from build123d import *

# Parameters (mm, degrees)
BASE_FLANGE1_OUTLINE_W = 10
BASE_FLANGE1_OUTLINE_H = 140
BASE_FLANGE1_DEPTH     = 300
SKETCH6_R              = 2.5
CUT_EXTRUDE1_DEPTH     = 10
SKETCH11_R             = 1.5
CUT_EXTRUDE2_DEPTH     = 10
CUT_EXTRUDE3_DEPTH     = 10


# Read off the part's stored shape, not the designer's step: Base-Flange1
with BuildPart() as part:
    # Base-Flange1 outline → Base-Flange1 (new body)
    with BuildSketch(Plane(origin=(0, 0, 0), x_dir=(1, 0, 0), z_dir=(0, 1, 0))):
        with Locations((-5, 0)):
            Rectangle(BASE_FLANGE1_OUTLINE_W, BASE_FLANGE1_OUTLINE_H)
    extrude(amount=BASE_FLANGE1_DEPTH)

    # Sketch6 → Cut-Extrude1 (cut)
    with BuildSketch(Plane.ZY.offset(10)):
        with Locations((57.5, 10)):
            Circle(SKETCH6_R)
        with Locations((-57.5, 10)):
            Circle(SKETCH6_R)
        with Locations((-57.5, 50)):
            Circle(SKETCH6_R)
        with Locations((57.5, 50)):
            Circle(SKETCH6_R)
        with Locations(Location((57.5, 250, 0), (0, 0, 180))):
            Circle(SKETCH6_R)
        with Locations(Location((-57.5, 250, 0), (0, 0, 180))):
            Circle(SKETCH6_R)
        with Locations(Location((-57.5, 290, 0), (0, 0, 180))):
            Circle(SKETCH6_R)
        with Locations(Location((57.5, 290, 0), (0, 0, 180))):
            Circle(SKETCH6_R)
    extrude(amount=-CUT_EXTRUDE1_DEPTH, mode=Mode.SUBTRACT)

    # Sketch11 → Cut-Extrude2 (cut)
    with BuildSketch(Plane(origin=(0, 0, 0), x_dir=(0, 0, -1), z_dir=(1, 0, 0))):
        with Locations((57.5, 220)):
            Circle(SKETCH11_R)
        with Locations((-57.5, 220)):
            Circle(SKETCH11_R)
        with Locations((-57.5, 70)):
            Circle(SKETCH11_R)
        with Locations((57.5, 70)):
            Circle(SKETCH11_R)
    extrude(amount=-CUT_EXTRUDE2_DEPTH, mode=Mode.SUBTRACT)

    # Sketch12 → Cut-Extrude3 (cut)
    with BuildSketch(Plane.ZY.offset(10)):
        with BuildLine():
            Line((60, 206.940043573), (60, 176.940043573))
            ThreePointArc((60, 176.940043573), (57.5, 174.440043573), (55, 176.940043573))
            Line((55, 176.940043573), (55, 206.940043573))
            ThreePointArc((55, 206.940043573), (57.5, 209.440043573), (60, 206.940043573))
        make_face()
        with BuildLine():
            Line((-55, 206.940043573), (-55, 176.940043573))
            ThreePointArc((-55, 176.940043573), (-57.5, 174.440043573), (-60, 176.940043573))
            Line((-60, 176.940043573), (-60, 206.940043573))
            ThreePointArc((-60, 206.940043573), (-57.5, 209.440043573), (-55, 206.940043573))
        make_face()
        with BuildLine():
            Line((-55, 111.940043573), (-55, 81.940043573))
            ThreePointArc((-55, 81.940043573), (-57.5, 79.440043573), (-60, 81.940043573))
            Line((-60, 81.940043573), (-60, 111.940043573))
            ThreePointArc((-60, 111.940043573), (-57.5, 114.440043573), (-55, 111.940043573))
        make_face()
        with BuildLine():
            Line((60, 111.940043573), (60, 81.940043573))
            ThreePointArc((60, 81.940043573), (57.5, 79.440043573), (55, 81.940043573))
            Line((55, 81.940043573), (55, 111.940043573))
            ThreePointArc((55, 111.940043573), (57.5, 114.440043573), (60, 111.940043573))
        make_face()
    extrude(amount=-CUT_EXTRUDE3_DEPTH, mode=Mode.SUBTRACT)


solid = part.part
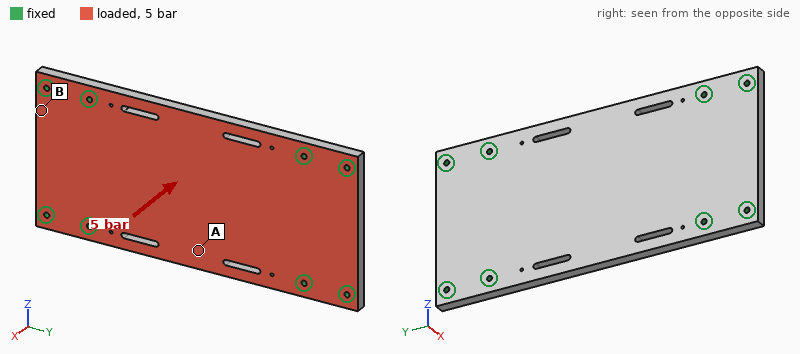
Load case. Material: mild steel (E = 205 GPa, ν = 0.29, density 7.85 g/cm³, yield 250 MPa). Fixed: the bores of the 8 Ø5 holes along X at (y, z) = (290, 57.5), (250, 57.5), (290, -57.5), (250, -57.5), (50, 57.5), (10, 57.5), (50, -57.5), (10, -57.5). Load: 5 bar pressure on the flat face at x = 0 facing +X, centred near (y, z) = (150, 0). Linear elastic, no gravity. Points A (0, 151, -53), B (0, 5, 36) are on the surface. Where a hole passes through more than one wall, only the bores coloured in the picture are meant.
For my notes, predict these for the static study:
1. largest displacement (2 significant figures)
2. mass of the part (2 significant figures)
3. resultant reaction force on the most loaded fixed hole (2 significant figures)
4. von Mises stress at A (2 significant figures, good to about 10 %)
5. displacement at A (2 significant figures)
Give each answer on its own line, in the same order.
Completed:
0.18 mm
3.2 kg
5.3 kN
56 MPa
0.17 mm
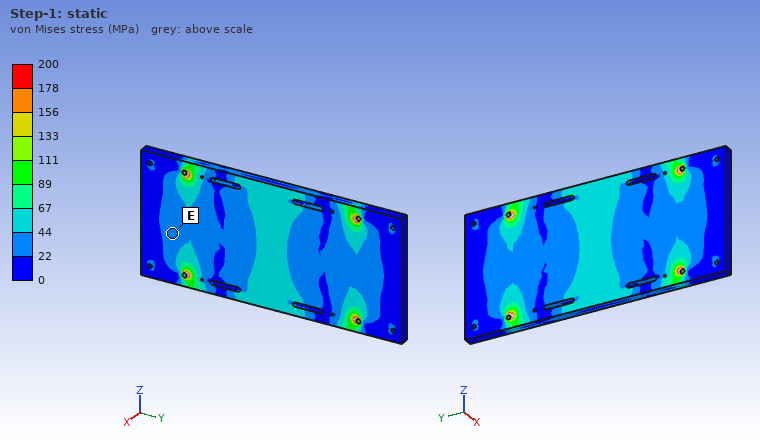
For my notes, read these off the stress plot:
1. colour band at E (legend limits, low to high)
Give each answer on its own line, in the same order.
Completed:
22 to 44 MPa
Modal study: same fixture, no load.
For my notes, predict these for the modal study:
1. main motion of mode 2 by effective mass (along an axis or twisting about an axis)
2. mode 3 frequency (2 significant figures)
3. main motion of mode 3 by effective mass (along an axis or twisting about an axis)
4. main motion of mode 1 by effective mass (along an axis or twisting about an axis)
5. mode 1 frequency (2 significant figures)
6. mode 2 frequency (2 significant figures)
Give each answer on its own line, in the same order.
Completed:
twisting about Y
2700 Hz
twisting about Z
along X
1100 Hz
1700 Hz
